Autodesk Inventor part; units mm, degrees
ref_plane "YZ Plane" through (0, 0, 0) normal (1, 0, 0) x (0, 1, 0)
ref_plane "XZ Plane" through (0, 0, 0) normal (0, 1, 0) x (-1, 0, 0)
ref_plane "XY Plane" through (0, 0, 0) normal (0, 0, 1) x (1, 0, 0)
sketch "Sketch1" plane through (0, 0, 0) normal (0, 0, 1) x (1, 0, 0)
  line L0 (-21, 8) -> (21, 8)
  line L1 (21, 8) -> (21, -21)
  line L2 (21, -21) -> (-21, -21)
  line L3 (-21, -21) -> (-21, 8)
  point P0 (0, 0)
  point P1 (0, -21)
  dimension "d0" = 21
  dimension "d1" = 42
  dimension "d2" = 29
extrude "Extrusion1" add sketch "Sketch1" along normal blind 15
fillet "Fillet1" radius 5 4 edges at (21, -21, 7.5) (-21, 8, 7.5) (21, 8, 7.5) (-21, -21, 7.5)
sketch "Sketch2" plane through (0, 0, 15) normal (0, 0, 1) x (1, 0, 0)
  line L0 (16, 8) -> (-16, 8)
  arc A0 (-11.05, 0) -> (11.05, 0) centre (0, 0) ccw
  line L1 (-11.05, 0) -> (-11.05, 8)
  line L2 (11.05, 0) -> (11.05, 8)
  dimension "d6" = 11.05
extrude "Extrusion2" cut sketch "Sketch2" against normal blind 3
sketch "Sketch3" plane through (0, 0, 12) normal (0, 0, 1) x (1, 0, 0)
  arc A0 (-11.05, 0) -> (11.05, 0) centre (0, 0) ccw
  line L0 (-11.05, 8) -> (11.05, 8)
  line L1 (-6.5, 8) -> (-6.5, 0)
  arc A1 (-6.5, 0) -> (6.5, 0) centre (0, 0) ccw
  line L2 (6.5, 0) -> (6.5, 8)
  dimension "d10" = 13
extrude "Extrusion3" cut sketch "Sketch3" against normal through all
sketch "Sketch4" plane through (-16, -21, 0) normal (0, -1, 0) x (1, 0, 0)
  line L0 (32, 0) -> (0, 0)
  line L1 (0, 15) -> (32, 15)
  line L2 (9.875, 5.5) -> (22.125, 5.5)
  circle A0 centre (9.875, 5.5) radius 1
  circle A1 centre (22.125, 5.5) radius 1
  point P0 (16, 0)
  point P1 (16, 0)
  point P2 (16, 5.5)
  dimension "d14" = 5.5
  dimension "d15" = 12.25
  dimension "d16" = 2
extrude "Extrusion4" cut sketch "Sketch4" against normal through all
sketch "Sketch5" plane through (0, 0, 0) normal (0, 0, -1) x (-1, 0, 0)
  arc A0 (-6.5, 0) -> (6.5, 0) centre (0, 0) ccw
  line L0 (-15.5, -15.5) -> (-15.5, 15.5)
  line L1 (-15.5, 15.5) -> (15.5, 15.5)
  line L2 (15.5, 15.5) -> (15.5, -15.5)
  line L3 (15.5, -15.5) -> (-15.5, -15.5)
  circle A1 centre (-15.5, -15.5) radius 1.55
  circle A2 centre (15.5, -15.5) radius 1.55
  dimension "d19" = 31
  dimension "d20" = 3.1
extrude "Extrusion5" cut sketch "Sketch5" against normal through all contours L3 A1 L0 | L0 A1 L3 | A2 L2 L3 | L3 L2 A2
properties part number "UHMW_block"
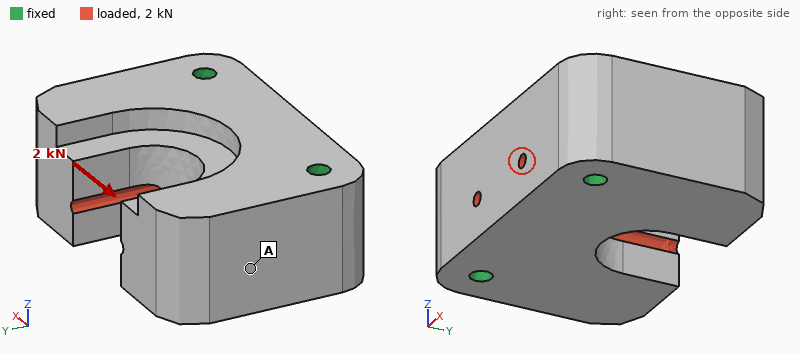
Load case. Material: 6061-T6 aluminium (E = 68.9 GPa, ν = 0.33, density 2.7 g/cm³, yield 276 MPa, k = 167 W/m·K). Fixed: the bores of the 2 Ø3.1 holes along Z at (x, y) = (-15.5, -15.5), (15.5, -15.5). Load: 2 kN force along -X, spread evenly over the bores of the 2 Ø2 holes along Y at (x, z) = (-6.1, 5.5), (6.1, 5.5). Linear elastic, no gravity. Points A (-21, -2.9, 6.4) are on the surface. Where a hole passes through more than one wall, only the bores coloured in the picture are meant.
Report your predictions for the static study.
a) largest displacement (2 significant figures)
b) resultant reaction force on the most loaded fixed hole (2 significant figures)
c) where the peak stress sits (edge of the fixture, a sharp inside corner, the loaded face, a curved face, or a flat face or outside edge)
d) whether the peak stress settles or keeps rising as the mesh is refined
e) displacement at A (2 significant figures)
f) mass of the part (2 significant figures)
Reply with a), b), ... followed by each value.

a) 3.8 µm
b) 1.1 kN
c) a sharp inside corner
d) keeps rising
e) 2.0 µm
f) 39 g
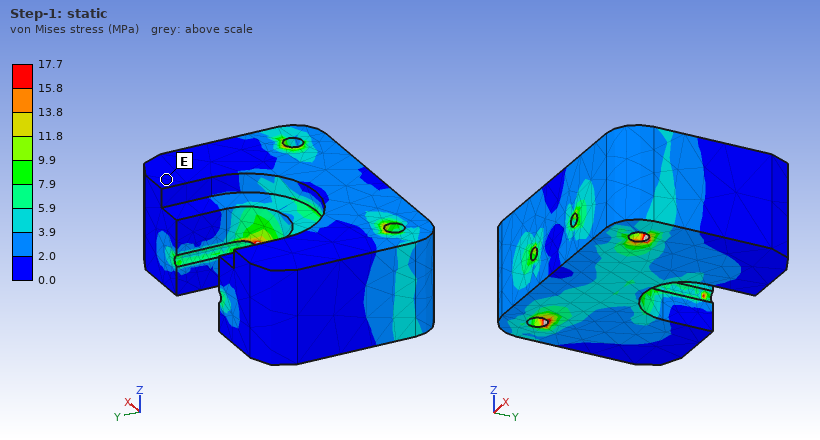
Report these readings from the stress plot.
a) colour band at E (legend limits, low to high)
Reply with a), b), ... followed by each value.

a) 0.0 to 2.0 MPa
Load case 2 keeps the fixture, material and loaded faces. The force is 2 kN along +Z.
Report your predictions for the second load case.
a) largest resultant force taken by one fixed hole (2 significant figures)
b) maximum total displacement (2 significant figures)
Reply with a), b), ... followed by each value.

a) 1.0 kN
b) 8.7 µm
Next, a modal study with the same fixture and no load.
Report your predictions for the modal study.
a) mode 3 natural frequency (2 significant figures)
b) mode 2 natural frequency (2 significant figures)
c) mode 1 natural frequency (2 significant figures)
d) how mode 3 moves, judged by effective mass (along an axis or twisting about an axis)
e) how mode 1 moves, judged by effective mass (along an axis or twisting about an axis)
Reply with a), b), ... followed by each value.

a) 19 kHz
b) 17 kHz
c) 16 kHz
d) twisting about Y
e) along Z
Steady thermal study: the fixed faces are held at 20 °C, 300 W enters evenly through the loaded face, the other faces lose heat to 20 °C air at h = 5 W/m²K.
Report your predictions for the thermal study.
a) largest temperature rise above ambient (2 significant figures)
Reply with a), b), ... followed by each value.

a) 55 K
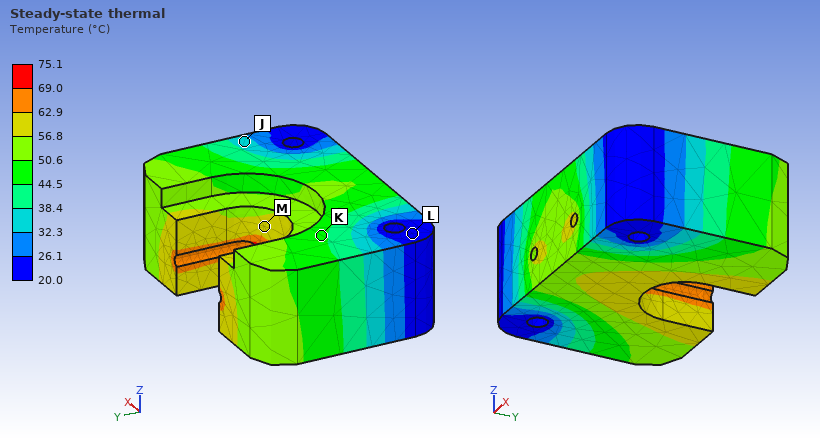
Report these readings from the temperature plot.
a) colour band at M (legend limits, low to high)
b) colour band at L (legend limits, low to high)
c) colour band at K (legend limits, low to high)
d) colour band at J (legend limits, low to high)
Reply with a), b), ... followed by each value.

a) 56.8 to 62.9 °C
b) 20.0 to 26.1 °C
c) 44.5 to 50.6 °C
d) 32.3 to 38.4 °C
